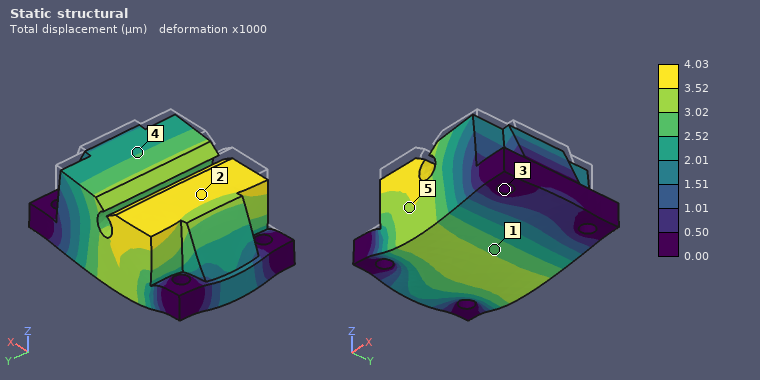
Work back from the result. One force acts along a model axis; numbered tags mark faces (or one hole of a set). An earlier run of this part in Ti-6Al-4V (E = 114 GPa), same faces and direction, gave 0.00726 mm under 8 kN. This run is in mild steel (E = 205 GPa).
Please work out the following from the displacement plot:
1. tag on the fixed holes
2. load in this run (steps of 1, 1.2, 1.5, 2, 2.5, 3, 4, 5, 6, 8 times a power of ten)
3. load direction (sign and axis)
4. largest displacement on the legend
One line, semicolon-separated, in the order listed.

3; 8 kN; -Z; 4.03 µm
